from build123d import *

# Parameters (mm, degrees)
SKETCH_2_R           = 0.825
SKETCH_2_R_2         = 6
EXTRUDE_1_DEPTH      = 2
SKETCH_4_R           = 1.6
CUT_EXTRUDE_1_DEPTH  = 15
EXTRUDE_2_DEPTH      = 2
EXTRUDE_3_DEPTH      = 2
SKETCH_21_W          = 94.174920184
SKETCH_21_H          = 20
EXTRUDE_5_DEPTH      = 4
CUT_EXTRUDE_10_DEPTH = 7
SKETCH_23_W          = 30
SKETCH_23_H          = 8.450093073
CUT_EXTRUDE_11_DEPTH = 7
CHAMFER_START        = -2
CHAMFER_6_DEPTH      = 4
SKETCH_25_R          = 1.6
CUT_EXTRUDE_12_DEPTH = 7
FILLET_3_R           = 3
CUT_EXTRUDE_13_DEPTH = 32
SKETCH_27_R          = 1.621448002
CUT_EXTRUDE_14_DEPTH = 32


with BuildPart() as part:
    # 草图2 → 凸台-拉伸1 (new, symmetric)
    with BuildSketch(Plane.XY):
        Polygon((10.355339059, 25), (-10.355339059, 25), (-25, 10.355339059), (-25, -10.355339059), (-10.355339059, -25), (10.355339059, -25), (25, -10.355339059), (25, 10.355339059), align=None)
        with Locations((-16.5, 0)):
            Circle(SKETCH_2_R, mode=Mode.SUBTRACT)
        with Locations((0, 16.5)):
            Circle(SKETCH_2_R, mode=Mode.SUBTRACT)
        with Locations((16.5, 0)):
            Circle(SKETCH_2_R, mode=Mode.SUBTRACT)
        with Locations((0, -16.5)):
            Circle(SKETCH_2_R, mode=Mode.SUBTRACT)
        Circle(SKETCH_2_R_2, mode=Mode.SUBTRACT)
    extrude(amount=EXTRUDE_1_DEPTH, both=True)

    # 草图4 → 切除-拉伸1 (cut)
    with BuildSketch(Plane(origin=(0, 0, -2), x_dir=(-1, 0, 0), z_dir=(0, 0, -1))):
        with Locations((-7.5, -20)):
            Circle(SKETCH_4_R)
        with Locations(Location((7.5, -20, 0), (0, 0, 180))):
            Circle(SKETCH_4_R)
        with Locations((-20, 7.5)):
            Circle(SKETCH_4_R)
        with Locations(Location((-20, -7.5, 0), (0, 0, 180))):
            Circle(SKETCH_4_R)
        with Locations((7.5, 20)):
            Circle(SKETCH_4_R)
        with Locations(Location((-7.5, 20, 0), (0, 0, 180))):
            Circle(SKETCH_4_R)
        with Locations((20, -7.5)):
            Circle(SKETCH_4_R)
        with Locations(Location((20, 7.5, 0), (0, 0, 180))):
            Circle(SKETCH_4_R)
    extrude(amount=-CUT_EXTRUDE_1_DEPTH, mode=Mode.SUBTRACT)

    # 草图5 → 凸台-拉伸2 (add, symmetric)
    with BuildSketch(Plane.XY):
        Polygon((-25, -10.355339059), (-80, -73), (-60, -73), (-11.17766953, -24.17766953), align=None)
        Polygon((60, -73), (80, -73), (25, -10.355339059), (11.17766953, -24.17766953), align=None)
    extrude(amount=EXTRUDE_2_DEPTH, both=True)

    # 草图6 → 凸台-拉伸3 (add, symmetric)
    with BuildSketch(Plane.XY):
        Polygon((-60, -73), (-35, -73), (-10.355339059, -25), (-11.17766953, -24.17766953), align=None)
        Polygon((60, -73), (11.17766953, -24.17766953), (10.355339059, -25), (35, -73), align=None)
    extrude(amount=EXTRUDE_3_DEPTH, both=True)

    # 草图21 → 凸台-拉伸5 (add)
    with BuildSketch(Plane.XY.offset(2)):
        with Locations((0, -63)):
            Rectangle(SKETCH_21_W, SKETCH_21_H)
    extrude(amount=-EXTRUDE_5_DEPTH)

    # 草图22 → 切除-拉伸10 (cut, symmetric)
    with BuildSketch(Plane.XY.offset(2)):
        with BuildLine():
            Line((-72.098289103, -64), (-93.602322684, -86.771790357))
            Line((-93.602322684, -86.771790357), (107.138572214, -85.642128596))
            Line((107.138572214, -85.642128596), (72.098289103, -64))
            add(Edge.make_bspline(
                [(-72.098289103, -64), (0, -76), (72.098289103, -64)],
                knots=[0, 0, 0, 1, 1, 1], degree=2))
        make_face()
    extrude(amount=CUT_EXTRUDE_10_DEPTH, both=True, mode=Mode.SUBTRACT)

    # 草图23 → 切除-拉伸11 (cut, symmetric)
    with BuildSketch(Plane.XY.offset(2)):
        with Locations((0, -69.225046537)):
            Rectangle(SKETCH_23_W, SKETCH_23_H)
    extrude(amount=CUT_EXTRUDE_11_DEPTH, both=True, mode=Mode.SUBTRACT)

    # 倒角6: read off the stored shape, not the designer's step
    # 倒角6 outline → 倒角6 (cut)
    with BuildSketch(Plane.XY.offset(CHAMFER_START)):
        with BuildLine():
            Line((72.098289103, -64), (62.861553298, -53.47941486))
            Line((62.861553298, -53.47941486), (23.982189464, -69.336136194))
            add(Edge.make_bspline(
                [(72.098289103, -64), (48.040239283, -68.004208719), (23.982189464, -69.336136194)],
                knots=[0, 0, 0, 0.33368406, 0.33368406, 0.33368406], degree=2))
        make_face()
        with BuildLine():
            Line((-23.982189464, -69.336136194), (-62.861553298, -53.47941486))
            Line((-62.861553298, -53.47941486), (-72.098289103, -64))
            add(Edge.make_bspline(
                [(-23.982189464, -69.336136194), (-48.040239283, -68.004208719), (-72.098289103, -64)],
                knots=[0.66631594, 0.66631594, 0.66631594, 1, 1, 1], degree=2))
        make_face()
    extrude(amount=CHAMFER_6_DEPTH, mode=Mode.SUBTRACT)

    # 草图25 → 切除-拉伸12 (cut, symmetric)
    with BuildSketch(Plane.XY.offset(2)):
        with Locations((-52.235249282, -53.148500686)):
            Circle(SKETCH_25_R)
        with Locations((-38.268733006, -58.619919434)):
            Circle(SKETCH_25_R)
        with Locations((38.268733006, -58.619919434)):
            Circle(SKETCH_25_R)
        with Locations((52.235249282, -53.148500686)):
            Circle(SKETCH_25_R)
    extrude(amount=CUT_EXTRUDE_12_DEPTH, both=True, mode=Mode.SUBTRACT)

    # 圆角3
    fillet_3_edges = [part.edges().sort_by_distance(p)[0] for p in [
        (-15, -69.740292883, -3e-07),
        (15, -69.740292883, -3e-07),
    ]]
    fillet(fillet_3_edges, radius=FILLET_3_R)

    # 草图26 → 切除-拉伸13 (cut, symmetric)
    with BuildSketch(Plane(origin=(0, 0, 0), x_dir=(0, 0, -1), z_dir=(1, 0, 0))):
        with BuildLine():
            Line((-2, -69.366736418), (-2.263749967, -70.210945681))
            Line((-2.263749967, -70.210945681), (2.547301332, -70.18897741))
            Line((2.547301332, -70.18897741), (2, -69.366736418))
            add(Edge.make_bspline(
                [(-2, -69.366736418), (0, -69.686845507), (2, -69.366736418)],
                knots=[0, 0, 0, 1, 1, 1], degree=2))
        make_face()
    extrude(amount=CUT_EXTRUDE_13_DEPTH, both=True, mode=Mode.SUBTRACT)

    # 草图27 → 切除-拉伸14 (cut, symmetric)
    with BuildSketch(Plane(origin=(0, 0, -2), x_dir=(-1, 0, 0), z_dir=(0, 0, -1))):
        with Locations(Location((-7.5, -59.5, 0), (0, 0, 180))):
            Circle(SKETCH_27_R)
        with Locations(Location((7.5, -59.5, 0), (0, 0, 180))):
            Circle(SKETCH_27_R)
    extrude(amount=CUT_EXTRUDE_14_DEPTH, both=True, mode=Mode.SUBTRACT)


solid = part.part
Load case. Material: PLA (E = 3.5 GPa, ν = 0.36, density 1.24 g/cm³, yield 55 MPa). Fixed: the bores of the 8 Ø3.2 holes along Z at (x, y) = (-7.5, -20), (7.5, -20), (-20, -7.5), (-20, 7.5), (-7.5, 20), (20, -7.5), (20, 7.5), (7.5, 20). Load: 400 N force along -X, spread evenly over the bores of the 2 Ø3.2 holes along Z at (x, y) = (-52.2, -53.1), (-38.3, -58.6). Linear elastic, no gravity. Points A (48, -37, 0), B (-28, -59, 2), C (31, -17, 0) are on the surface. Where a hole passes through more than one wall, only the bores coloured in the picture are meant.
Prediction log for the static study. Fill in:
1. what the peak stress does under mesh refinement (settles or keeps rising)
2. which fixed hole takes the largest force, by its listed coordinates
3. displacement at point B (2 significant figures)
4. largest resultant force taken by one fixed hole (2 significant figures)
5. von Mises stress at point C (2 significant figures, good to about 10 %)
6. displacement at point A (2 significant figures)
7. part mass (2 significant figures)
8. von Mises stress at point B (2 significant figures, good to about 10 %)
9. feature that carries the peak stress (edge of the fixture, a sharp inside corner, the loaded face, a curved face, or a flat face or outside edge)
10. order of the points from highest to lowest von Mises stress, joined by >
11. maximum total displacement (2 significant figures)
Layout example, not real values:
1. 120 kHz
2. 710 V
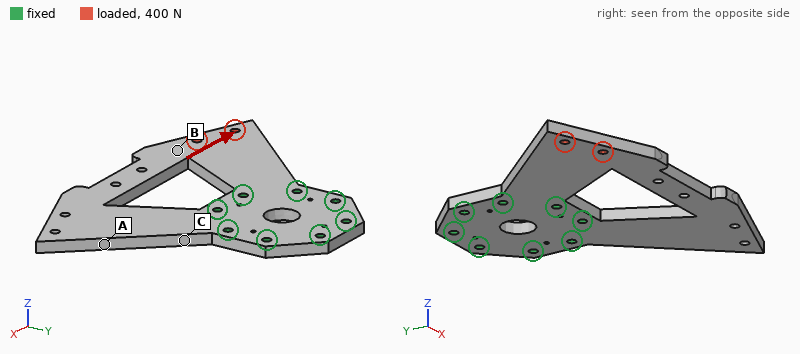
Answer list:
1. keeps rising
2. (-7.5, -20)
3. 0.49 mm
4. 480 N
5. 14 MPa
6. 0.35 mm
7. 27 g
8. 5.6 MPa
9. a sharp inside corner
10. C > B > A
11. 0.71 mm
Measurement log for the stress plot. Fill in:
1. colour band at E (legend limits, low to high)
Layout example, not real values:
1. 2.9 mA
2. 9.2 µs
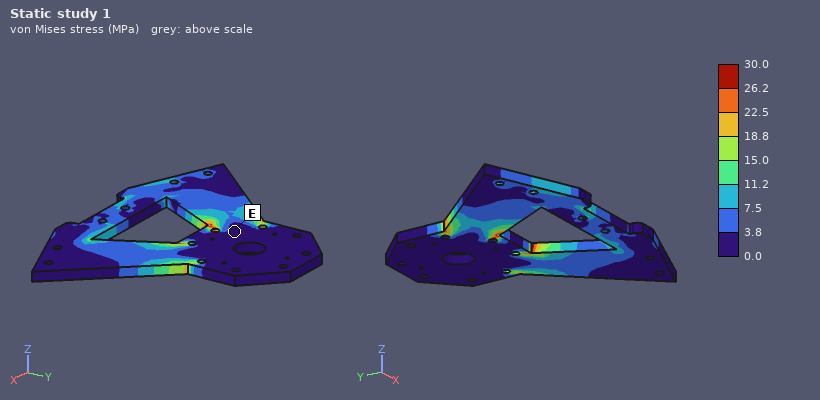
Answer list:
1. 0.0 to 3.8 MPa
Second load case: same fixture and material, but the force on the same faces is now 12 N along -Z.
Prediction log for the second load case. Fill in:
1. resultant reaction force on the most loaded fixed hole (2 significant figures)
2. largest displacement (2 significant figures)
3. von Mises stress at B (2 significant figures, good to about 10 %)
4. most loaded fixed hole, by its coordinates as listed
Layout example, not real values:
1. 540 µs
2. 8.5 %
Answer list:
1. 14 N
2. 1.4 mm
3. 1.7 MPa
4. (-7.5, -20)
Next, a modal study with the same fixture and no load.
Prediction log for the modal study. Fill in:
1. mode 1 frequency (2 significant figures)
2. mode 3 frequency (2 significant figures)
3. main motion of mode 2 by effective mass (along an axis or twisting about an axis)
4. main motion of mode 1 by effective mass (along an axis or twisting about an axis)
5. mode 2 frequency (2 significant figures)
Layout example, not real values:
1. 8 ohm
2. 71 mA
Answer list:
1. 260 Hz
2. 710 Hz
3. twisting about Y
4. along Z
5. 310 Hz
